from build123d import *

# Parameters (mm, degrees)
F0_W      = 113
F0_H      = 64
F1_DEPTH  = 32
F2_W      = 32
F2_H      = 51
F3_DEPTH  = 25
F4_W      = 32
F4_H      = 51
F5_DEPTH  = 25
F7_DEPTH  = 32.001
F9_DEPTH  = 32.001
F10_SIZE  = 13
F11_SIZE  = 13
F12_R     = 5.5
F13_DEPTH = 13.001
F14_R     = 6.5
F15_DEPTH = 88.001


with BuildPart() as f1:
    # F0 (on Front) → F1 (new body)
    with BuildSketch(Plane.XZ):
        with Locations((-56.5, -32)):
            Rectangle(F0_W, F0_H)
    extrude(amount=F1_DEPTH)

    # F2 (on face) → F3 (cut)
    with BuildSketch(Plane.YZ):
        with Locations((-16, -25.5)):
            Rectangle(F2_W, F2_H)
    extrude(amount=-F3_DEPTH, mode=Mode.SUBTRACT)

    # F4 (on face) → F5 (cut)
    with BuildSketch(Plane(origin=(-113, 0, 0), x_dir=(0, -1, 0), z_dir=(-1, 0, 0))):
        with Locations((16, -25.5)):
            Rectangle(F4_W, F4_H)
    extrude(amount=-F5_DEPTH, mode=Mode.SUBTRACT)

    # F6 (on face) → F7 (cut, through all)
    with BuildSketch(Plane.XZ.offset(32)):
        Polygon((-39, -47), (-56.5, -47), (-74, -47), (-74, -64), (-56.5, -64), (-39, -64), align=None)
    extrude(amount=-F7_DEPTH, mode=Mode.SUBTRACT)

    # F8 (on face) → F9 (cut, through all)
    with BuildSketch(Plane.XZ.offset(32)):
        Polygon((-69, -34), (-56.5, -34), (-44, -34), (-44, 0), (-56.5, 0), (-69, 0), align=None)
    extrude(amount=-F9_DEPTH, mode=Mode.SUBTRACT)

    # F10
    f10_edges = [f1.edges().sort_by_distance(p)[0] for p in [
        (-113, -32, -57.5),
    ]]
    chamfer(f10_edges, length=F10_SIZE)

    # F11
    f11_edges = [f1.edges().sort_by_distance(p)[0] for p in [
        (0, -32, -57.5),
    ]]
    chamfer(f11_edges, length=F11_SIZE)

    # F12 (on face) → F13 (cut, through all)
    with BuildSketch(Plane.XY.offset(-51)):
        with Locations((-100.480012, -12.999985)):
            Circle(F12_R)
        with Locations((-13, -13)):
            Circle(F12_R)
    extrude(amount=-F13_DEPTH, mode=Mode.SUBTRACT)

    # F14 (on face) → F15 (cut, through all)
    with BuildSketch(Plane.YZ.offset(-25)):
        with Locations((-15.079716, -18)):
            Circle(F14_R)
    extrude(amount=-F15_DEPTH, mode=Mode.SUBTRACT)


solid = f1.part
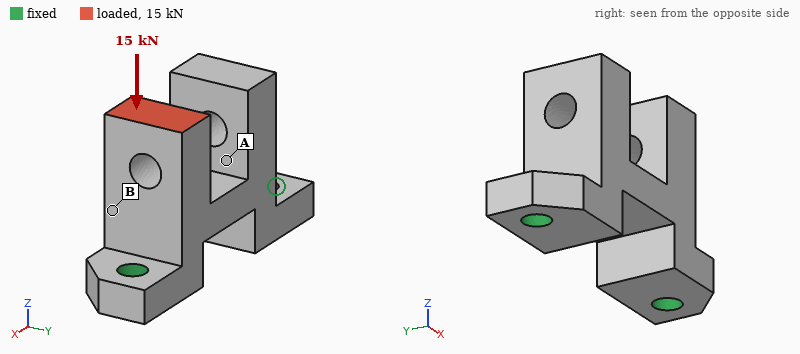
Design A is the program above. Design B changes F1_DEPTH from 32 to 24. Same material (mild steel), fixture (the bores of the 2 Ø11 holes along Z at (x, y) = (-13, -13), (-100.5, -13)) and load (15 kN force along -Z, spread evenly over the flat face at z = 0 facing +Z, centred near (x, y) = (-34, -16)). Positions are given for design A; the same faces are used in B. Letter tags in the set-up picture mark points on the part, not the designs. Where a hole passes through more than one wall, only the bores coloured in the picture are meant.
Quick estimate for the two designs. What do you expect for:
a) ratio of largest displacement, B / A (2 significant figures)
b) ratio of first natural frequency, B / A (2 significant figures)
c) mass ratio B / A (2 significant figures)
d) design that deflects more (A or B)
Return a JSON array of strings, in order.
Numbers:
["1.2", "0.98", "0.72", "B"]
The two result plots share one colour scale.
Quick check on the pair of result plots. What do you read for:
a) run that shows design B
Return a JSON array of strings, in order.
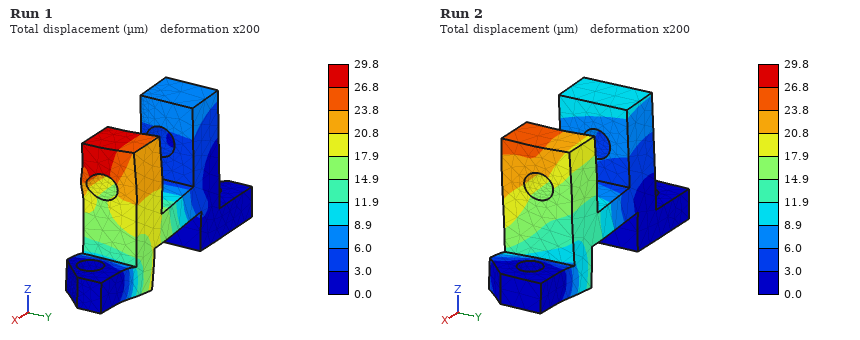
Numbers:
["Run 1"]
